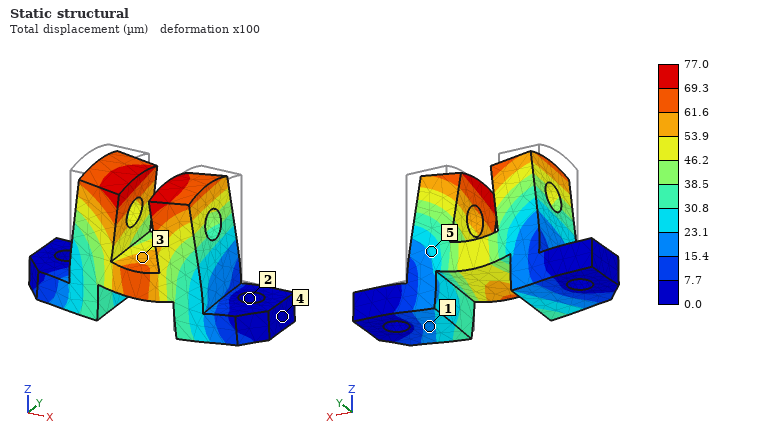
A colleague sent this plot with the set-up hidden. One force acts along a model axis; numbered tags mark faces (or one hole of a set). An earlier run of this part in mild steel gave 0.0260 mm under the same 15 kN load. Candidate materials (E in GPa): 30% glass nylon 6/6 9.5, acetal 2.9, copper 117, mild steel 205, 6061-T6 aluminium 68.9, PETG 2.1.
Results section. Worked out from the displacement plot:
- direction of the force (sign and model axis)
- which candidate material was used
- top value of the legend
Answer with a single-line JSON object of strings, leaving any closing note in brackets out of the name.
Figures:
{"direction of the force": "-Z", "which candidate material was used": "6061-T6 aluminium", "top value of the legend": "77.0 µm"}
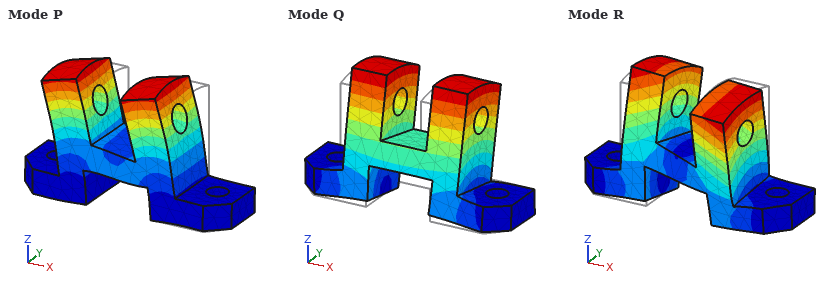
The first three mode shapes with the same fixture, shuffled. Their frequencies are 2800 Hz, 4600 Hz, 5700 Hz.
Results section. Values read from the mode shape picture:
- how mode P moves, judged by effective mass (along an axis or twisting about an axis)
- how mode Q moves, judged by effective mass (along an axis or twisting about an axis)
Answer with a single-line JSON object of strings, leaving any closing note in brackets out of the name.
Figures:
{"how mode P moves, judged by effective mass": "along X", "how mode Q moves, judged by effective mass": "along Y"}
